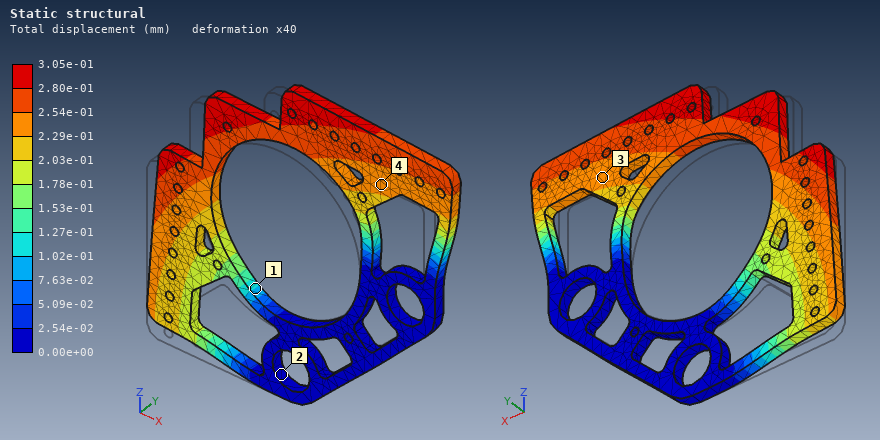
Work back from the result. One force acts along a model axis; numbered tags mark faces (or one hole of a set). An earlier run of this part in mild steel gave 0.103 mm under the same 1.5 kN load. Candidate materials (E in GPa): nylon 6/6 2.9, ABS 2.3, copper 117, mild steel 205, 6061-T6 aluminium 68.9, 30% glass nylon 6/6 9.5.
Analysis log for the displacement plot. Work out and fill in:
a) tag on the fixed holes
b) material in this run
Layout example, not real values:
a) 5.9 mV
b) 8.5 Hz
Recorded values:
a) 2
b) 6061-T6 aluminium
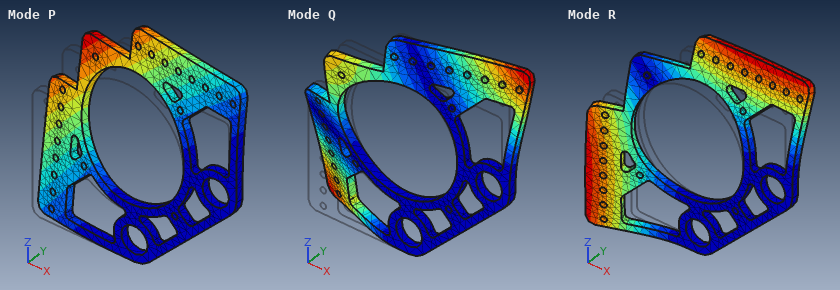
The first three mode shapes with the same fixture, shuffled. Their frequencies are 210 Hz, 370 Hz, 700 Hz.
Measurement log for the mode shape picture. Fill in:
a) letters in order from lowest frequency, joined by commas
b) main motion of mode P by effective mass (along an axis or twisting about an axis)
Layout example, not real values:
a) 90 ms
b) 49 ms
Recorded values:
a) P, R, Q
b) along Y
